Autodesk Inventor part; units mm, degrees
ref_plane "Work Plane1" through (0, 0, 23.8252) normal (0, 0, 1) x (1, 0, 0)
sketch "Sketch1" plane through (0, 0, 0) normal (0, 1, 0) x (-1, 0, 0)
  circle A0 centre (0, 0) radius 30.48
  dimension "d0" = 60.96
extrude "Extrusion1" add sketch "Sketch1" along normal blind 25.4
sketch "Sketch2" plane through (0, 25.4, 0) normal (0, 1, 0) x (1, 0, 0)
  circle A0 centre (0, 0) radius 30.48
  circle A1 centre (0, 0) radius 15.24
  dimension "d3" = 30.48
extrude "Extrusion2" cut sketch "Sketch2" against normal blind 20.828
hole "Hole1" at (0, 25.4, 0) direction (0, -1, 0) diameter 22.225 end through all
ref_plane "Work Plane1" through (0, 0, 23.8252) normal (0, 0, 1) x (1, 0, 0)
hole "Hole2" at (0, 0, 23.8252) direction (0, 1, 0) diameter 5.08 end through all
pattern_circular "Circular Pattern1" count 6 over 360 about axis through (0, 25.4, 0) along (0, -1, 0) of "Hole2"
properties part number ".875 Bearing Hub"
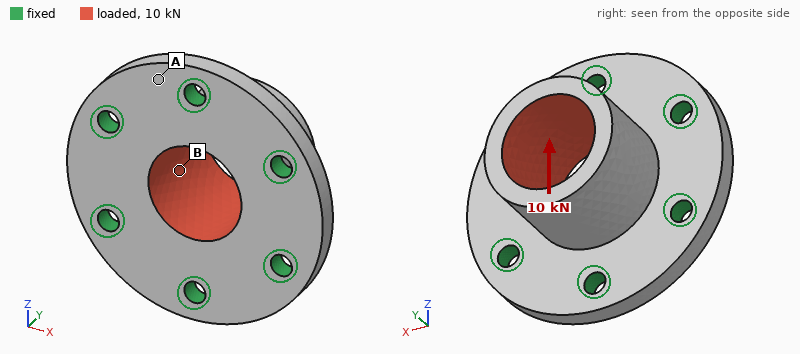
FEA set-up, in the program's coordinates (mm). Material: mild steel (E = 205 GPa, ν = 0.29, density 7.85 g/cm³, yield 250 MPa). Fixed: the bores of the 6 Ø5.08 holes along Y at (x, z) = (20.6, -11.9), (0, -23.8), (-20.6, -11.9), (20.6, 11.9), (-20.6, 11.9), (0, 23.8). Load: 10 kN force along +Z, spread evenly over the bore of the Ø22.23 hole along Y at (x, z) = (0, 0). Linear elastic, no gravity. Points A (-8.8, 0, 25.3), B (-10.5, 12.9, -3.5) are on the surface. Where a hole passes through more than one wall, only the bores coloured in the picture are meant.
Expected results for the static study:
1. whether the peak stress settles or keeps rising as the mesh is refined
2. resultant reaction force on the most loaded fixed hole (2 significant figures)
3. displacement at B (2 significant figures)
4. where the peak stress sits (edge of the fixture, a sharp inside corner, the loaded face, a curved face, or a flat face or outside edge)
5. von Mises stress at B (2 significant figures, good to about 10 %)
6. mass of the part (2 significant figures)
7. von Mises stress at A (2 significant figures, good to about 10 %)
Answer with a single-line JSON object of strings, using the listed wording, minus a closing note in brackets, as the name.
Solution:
{"whether the peak stress settles or keeps rising as the mesh is refined": "keeps rising", "resultant reaction force on the most loaded fixed hole": "2.9 kN", "displacement at B": "9.9 µm", "where the peak stress sits": "edge of the fixture", "von Mises stress at B": "59 MPa", "mass of the part": "140 g", "von Mises stress at A": "25 MPa"}
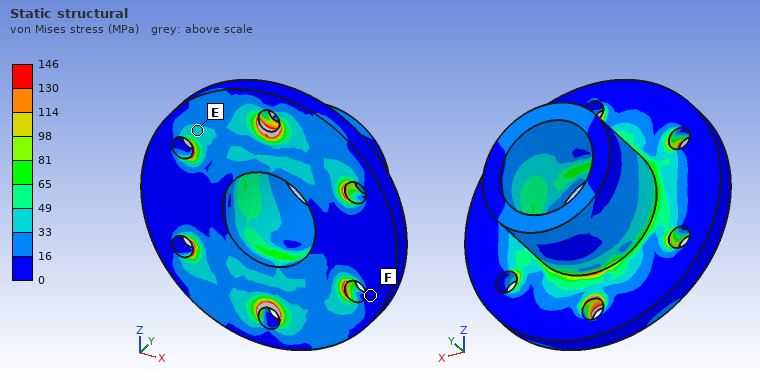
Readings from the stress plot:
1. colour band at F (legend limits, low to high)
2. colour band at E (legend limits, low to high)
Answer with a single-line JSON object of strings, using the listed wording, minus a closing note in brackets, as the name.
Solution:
{"colour band at F": "0 to 16 MPa", "colour band at E": "33 to 49 MPa"}
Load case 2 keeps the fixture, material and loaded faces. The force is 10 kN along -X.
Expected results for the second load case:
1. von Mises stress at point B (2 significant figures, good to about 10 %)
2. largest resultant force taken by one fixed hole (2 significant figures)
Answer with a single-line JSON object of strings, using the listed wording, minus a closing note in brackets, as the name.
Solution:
{"von Mises stress at point B": "27 MPa", "largest resultant force taken by one fixed hole": "2.6 kN"}
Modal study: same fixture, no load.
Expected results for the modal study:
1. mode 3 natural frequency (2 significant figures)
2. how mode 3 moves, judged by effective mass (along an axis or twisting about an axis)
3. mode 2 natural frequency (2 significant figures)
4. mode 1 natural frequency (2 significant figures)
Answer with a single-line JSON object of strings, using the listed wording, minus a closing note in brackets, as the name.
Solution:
{"mode 3 natural frequency": "18 kHz", "how mode 3 moves, judged by effective mass": "along Y", "mode 2 natural frequency": "14 kHz", "mode 1 natural frequency": "14 kHz"}
